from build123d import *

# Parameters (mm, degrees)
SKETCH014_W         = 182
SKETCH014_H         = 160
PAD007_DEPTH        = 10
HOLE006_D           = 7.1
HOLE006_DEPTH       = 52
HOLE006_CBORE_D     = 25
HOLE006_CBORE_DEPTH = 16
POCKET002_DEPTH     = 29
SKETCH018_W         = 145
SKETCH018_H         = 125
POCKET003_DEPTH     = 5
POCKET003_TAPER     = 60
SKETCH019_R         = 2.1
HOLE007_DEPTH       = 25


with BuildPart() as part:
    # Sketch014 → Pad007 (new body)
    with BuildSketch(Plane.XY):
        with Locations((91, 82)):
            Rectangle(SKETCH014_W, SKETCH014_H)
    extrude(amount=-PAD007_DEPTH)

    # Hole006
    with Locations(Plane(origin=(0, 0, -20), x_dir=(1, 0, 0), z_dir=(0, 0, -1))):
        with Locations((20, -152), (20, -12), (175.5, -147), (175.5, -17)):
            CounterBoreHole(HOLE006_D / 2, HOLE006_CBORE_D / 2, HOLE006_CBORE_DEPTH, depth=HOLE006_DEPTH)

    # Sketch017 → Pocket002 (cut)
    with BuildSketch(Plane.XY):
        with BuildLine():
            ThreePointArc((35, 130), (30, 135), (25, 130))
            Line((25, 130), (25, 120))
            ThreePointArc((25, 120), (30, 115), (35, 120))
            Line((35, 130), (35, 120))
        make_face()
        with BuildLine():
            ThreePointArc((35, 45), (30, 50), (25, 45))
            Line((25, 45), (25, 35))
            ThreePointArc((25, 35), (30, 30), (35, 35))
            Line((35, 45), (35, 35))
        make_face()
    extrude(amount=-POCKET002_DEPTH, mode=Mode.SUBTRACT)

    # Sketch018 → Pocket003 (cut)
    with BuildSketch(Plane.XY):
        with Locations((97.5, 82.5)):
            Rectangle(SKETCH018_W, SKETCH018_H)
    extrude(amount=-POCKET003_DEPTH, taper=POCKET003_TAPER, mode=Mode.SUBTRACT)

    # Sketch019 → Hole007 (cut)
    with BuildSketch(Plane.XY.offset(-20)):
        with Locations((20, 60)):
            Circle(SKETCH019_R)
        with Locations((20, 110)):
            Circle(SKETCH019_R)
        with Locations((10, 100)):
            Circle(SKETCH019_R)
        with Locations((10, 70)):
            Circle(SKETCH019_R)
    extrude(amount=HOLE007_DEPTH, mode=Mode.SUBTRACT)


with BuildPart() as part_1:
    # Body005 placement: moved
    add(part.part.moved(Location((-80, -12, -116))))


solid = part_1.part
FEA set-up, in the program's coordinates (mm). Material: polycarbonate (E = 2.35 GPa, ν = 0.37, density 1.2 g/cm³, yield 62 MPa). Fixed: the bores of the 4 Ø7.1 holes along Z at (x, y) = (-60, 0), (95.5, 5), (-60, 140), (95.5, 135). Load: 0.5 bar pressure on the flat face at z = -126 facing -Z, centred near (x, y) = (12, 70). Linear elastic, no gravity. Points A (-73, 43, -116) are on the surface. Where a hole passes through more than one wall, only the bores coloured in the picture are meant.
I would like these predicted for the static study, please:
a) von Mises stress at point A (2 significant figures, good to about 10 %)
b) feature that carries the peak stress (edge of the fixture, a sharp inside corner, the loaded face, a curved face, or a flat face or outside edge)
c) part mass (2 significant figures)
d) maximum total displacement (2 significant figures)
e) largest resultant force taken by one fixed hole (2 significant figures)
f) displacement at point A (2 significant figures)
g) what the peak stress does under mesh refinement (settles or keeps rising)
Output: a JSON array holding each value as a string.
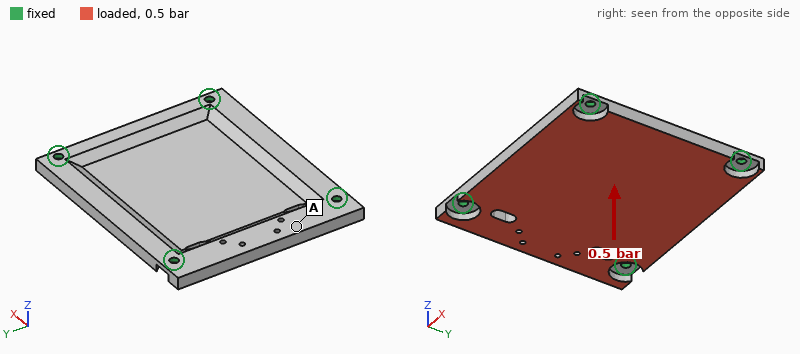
["4.5 MPa", "edge of the fixture", "240 g", "2.8 mm", "1.1 kN", "0.55 mm", "keeps rising"]
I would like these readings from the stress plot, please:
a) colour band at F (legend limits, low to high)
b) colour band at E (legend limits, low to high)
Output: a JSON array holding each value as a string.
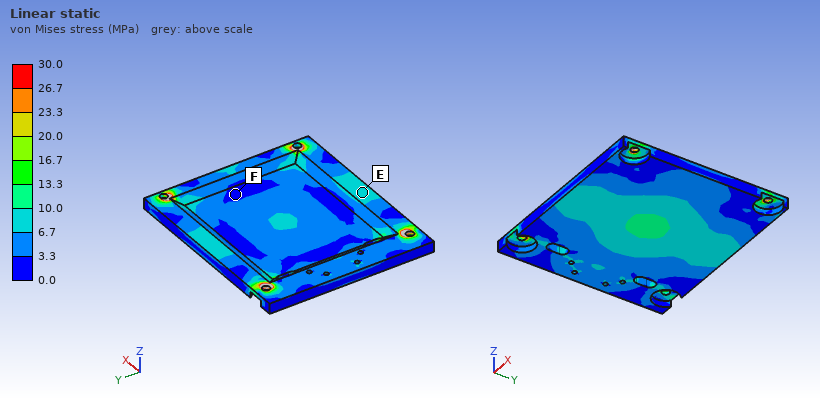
["0.0 to 3.3 MPa", "6.7 to 10.0 MPa"]
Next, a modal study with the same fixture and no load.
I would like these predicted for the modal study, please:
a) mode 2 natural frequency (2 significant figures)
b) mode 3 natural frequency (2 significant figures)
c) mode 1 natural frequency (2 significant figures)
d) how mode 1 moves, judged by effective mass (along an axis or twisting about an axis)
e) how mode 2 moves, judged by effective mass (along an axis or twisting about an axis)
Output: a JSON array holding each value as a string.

["450 Hz", "490 Hz", "330 Hz", "along Z", "twisting about X"]
